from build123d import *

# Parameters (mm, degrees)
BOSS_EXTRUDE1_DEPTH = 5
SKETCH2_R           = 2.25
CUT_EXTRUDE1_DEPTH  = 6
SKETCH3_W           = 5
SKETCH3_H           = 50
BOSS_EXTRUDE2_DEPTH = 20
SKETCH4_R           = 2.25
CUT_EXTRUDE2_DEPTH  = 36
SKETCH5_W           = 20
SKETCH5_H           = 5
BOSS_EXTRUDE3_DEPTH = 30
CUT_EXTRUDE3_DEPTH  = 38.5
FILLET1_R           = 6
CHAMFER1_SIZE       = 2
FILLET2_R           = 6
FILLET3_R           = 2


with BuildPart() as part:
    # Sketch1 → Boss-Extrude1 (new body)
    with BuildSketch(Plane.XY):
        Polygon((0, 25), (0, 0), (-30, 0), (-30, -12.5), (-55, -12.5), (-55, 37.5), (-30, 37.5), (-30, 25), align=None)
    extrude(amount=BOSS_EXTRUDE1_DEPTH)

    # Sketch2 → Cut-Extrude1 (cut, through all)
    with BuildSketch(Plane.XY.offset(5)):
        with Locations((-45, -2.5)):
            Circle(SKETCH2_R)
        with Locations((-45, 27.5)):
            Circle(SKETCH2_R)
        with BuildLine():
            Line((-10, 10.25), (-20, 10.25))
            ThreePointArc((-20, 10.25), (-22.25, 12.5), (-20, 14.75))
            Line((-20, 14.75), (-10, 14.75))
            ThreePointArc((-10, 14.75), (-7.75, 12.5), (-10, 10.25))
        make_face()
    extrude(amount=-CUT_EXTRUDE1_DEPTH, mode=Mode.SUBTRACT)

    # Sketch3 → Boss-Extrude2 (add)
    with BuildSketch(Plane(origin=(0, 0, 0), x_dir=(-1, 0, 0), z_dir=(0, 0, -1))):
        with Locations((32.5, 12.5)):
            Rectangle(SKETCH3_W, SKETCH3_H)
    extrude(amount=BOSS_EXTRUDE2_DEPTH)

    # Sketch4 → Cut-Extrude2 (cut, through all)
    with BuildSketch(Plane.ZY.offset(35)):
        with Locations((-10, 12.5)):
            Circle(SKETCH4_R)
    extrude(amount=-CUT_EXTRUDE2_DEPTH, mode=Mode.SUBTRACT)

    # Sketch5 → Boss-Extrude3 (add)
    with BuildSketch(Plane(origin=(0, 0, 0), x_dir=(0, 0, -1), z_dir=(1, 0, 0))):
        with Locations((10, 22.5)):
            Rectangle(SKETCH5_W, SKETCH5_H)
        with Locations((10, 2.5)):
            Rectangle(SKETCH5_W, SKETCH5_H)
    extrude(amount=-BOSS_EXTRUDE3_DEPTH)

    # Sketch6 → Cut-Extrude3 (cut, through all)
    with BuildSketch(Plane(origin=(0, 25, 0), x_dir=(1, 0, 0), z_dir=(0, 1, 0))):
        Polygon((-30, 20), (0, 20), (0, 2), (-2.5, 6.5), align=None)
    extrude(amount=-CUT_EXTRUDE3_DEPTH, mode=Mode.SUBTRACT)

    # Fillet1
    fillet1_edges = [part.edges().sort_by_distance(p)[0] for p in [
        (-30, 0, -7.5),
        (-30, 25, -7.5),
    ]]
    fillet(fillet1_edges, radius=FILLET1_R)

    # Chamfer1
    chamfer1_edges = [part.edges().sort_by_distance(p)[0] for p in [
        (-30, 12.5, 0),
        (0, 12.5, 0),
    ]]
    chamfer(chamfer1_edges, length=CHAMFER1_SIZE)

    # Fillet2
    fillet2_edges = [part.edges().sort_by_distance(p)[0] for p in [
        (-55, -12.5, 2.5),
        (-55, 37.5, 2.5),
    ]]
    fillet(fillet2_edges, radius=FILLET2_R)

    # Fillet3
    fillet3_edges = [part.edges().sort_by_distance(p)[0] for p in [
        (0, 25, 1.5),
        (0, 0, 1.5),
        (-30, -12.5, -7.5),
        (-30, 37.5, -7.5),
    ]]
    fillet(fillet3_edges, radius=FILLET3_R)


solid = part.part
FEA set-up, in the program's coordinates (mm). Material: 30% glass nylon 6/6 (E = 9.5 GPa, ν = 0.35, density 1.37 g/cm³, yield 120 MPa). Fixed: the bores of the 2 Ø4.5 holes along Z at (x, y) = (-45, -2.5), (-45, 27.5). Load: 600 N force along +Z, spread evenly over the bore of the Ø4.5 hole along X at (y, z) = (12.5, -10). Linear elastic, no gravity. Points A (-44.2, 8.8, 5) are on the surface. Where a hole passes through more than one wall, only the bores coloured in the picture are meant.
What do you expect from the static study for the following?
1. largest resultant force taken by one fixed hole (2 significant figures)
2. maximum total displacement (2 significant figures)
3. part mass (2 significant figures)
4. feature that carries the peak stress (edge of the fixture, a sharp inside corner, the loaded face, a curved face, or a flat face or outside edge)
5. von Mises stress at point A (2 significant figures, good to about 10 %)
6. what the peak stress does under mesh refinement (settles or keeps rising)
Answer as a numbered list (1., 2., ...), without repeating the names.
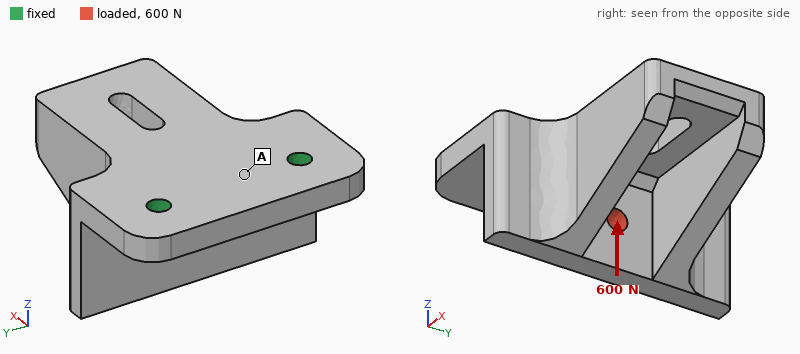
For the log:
1. 300 N
2. 0.44 mm
3. 25 g
4. edge of the fixture
5. 11 MPa
6. keeps rising
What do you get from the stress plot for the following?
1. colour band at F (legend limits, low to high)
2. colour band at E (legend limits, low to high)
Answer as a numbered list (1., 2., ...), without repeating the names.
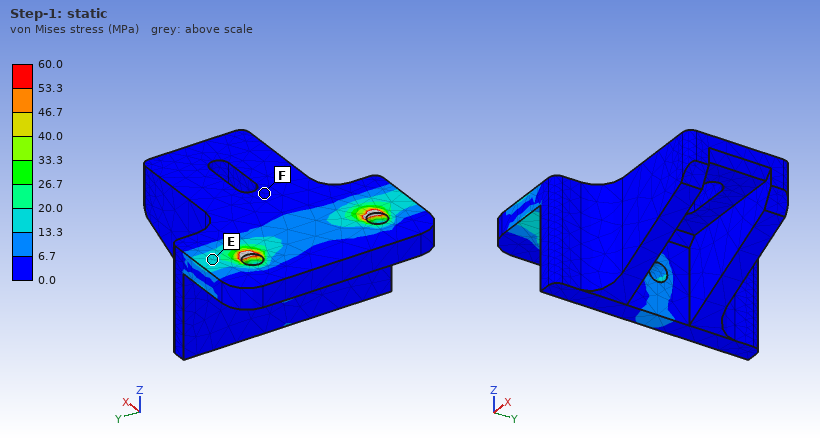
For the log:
1. 0.0 to 6.7 MPa
2. 13.3 to 20.0 MPa
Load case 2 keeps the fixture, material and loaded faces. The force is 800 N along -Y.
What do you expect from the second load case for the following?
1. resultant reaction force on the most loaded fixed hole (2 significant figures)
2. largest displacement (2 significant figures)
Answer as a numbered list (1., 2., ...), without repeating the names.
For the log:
1. 580 N
2. 0.13 mm
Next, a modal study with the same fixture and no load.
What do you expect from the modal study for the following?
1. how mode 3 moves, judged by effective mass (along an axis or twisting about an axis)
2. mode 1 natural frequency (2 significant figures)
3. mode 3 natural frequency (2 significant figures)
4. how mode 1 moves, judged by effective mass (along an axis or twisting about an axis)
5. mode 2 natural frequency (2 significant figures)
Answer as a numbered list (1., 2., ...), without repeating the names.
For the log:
1. along Y
2. 1100 Hz
3. 4800 Hz
4. along Z
5. 3500 Hz
